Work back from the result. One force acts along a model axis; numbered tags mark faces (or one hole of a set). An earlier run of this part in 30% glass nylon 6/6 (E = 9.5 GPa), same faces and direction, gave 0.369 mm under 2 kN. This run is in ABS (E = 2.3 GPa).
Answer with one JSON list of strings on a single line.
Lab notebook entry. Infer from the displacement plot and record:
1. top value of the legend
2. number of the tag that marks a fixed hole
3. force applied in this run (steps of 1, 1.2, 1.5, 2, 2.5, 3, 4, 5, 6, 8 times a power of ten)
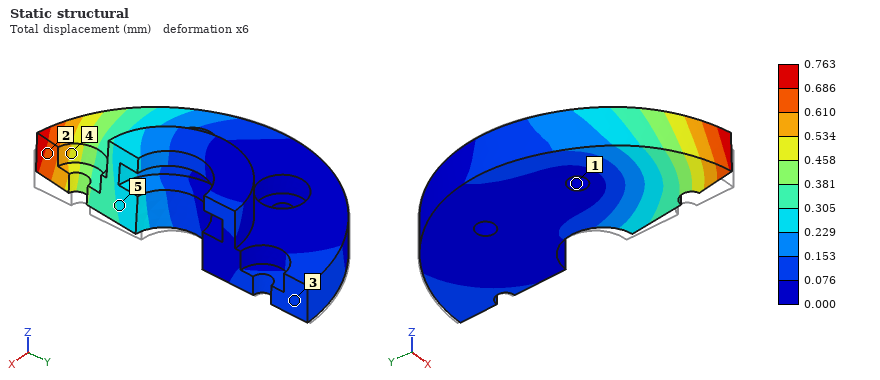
["0.763 mm", "1", "1 kN"]
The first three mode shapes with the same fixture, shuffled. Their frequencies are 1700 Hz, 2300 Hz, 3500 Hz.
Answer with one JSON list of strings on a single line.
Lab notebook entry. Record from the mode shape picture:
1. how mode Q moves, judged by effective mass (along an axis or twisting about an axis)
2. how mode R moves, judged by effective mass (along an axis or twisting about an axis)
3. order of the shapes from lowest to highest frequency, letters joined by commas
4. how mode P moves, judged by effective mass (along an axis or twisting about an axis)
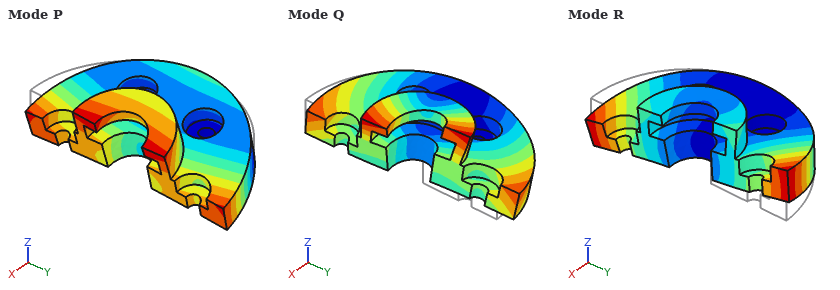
["along Y", "twisting about X", "P, R, Q", "along Z"]
